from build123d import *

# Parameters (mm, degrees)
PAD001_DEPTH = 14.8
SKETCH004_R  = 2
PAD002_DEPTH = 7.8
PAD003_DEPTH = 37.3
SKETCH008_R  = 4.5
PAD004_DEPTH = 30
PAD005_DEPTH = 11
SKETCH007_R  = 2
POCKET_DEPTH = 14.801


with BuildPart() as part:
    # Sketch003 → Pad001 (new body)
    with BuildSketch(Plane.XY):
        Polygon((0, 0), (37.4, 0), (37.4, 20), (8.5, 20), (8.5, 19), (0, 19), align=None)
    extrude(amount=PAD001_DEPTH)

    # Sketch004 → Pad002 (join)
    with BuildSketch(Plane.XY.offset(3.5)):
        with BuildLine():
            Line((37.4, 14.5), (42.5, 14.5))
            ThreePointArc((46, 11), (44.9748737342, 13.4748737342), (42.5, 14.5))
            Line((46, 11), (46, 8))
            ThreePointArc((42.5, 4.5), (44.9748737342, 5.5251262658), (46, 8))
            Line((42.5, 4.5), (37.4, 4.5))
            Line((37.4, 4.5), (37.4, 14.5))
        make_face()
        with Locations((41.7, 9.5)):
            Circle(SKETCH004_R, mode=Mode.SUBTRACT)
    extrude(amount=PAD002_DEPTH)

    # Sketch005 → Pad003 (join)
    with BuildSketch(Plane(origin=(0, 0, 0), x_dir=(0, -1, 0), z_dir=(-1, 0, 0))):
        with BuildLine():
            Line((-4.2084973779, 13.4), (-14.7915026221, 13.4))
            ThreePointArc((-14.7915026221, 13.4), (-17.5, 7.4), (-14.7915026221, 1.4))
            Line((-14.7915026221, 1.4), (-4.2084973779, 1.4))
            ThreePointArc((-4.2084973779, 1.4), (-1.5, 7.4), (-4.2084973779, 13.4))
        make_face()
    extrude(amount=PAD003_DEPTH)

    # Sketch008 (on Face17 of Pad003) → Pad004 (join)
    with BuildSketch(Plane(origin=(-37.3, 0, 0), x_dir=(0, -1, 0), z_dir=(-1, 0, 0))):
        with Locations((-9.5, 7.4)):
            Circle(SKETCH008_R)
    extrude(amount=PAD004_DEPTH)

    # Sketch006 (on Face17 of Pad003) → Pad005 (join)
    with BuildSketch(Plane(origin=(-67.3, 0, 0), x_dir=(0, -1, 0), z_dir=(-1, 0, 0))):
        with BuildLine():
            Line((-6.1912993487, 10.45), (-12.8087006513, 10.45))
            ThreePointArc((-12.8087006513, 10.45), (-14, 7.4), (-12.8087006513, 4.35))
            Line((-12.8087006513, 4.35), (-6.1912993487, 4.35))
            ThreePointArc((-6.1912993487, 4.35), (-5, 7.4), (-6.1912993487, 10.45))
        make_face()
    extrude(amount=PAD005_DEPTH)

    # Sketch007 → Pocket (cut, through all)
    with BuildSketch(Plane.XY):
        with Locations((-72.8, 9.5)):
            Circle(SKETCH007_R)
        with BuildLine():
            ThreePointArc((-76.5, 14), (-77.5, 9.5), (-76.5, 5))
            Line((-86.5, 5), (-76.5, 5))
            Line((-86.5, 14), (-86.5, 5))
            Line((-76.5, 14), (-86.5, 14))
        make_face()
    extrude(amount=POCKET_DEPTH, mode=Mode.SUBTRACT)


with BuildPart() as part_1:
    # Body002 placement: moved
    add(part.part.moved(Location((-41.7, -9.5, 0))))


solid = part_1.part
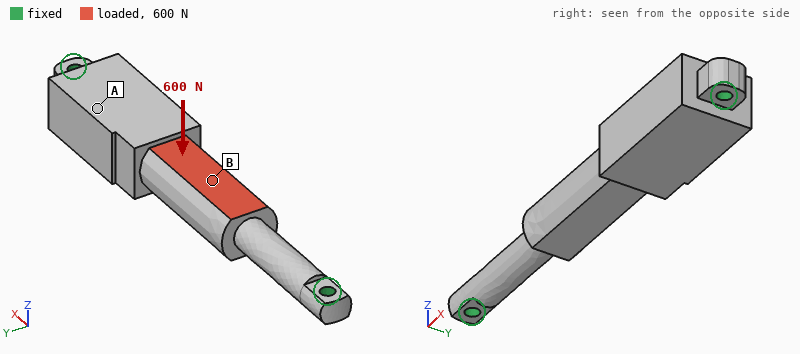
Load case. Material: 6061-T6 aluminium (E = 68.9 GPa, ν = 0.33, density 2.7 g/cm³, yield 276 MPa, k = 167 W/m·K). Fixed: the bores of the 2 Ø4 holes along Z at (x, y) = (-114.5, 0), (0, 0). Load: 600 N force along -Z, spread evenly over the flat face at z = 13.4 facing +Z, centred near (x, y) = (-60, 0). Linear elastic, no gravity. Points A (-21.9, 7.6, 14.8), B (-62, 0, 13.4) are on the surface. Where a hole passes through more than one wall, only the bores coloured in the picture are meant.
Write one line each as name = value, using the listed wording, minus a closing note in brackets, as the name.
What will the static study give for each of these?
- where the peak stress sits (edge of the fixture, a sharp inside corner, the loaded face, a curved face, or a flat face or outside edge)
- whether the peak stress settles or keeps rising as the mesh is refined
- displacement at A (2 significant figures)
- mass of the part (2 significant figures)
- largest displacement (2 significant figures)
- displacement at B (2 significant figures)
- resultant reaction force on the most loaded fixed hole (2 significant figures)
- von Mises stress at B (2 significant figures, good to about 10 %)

where the peak stress sits = edge of the fixture
whether the peak stress settles or keeps rising as the mesh is refined = keeps rising
displacement at A = 32 µm
mass of the part = 55 g
largest displacement = 84 µm
displacement at B = 82 µm
resultant reaction force on the most loaded fixed hole = 310 N
von Mises stress at B = 24 MPa
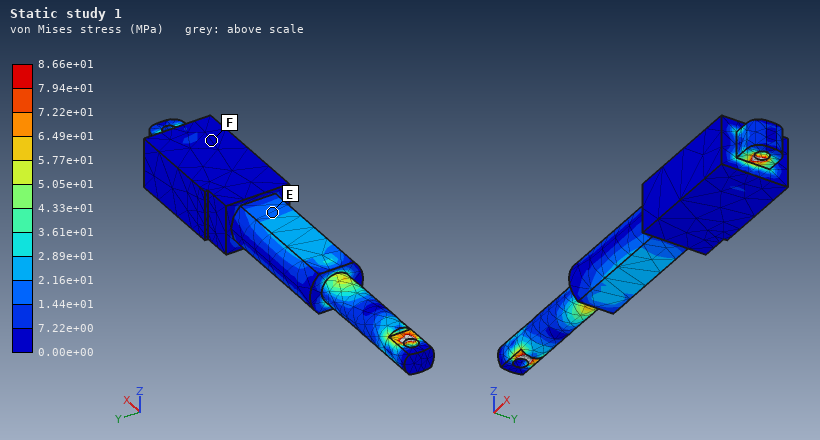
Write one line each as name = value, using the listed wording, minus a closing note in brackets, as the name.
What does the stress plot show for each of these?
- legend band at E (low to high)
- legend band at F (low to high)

legend band at E = 1.44e+01 to 2.16e+01 MPa
legend band at F = 0.00e+00 to 7.22e+00 MPa
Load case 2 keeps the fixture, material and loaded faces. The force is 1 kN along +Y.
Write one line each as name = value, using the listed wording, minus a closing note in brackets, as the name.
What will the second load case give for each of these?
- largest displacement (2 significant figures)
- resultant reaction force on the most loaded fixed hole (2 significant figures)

largest displacement = 0.13 mm
resultant reaction force on the most loaded fixed hole = 510 N
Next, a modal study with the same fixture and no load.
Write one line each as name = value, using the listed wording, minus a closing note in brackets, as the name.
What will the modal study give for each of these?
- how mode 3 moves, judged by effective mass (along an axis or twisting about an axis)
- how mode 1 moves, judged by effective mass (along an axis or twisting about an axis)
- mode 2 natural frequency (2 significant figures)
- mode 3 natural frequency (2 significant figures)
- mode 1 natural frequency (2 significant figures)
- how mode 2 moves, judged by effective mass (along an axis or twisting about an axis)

how mode 3 moves, judged by effective mass = twisting about X
how mode 1 moves, judged by effective mass = along Z
mode 2 natural frequency = 2900 Hz
mode 3 natural frequency = 7400 Hz
mode 1 natural frequency = 2700 Hz
how mode 2 moves, judged by effective mass = along Y
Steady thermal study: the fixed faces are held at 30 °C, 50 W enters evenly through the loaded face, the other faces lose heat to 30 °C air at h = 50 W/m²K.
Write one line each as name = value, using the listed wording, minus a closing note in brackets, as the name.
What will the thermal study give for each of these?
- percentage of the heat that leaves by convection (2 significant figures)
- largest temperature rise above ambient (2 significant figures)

percentage of the heat that leaves by convection = 16 %
largest temperature rise above ambient = 52 K
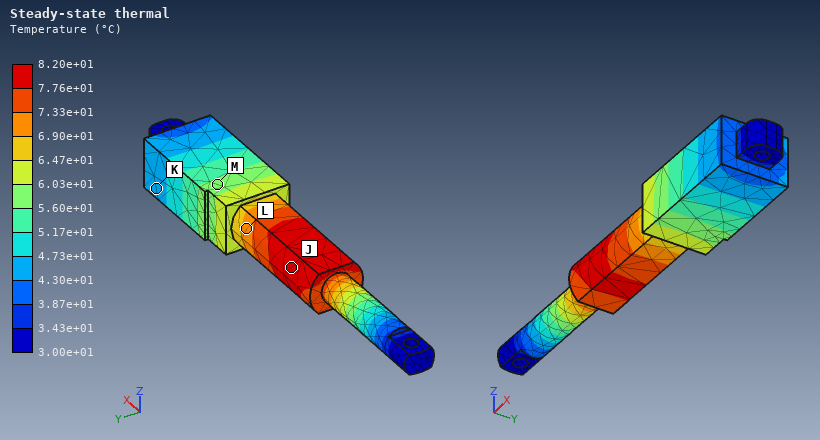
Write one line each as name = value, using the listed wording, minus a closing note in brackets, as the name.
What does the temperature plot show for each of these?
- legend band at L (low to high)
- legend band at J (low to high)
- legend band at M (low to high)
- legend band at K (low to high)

legend band at L = 6.90e+01 to 7.33e+01 °C
legend band at J = 7.76e+01 to 8.20e+01 °C
legend band at M = 5.60e+01 to 6.03e+01 °C
legend band at K = 4.30e+01 to 4.73e+01 °C
